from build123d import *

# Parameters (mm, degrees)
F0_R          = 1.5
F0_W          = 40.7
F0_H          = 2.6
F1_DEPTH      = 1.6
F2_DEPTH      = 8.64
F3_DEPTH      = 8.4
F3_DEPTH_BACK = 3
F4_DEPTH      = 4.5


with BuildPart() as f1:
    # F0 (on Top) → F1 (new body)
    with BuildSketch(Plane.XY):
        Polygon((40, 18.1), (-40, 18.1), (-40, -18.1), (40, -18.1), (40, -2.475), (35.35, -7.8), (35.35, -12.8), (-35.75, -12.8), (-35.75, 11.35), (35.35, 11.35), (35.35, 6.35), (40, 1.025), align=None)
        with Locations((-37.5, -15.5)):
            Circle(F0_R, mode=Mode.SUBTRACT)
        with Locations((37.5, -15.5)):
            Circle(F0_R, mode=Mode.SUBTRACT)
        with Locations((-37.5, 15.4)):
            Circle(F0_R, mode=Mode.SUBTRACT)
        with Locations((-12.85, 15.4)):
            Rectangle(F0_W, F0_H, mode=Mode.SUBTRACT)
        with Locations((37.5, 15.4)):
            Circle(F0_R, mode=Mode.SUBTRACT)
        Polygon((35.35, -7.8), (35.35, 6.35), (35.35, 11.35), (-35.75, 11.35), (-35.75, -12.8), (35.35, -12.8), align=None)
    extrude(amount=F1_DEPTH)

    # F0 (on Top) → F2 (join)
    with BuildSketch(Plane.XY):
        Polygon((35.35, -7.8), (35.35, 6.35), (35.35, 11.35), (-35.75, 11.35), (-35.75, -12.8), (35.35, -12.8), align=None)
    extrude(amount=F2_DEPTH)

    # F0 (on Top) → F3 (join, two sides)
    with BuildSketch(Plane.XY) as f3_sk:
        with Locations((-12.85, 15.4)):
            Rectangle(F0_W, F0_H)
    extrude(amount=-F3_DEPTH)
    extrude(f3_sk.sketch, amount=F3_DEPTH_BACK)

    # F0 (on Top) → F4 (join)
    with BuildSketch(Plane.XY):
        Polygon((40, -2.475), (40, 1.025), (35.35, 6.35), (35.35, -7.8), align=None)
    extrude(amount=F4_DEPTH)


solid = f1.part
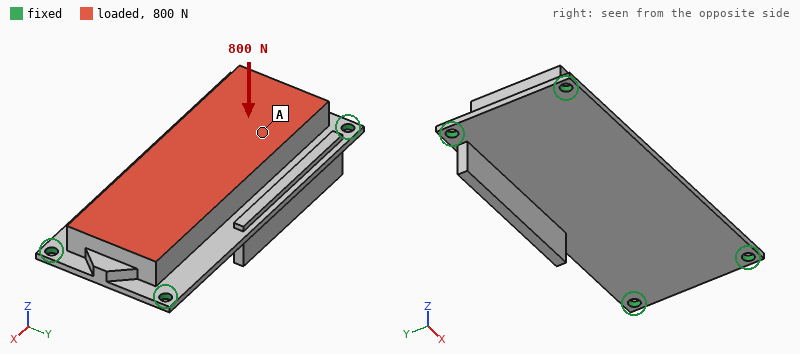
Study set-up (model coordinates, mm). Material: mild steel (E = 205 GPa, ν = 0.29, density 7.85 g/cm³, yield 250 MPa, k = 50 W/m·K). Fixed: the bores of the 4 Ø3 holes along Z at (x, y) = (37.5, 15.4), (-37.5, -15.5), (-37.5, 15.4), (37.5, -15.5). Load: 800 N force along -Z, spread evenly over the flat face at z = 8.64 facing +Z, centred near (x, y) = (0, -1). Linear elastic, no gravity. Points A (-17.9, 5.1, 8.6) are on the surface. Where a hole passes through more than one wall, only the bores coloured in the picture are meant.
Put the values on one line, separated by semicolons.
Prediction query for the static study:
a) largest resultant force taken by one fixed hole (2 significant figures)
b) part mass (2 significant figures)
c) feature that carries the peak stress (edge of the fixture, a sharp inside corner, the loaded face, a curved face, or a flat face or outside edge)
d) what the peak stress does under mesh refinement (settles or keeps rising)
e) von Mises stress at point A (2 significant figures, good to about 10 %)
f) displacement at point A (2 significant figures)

370 N; 140 g; edge of the fixture; keeps rising; 9.3 MPa; 9.4 µm
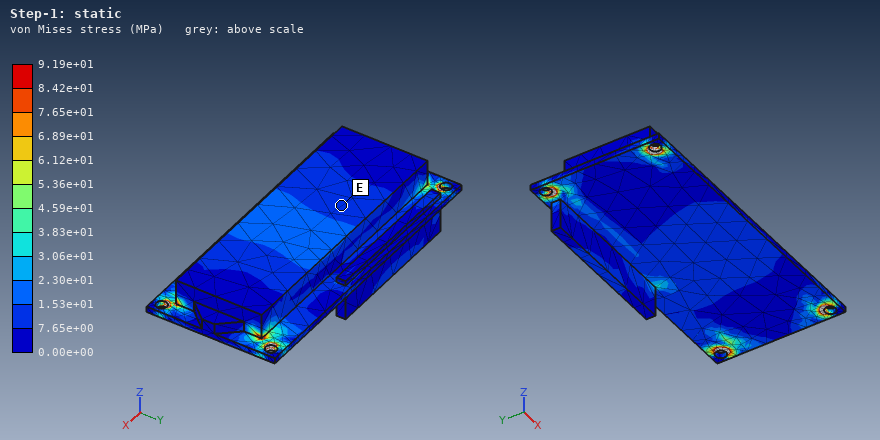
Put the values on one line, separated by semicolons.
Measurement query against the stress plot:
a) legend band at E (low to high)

7.65e+00 to 1.53e+01 MPa
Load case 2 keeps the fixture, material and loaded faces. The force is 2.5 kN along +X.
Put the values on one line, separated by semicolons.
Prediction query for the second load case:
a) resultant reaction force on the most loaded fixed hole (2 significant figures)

710 N
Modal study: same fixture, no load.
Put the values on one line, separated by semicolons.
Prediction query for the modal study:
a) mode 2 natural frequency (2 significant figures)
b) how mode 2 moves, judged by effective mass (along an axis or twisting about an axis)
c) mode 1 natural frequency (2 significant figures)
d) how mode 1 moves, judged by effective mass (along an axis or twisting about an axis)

6800 Hz; twisting about X; 3800 Hz; along Z
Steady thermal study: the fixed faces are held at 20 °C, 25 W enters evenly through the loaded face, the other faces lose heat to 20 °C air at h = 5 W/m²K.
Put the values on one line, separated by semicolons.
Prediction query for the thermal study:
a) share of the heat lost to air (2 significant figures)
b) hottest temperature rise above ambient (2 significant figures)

6.2 %; 60 K
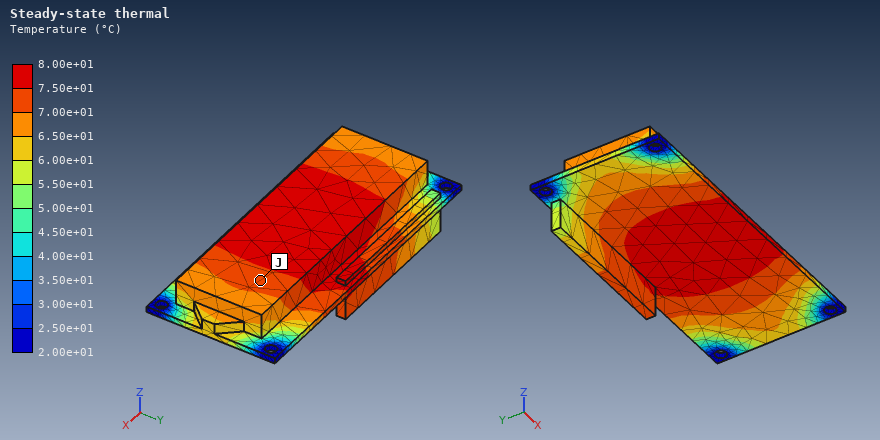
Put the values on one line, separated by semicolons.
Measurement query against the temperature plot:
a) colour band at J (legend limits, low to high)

7.00e+01 to 7.50e+01 °C
